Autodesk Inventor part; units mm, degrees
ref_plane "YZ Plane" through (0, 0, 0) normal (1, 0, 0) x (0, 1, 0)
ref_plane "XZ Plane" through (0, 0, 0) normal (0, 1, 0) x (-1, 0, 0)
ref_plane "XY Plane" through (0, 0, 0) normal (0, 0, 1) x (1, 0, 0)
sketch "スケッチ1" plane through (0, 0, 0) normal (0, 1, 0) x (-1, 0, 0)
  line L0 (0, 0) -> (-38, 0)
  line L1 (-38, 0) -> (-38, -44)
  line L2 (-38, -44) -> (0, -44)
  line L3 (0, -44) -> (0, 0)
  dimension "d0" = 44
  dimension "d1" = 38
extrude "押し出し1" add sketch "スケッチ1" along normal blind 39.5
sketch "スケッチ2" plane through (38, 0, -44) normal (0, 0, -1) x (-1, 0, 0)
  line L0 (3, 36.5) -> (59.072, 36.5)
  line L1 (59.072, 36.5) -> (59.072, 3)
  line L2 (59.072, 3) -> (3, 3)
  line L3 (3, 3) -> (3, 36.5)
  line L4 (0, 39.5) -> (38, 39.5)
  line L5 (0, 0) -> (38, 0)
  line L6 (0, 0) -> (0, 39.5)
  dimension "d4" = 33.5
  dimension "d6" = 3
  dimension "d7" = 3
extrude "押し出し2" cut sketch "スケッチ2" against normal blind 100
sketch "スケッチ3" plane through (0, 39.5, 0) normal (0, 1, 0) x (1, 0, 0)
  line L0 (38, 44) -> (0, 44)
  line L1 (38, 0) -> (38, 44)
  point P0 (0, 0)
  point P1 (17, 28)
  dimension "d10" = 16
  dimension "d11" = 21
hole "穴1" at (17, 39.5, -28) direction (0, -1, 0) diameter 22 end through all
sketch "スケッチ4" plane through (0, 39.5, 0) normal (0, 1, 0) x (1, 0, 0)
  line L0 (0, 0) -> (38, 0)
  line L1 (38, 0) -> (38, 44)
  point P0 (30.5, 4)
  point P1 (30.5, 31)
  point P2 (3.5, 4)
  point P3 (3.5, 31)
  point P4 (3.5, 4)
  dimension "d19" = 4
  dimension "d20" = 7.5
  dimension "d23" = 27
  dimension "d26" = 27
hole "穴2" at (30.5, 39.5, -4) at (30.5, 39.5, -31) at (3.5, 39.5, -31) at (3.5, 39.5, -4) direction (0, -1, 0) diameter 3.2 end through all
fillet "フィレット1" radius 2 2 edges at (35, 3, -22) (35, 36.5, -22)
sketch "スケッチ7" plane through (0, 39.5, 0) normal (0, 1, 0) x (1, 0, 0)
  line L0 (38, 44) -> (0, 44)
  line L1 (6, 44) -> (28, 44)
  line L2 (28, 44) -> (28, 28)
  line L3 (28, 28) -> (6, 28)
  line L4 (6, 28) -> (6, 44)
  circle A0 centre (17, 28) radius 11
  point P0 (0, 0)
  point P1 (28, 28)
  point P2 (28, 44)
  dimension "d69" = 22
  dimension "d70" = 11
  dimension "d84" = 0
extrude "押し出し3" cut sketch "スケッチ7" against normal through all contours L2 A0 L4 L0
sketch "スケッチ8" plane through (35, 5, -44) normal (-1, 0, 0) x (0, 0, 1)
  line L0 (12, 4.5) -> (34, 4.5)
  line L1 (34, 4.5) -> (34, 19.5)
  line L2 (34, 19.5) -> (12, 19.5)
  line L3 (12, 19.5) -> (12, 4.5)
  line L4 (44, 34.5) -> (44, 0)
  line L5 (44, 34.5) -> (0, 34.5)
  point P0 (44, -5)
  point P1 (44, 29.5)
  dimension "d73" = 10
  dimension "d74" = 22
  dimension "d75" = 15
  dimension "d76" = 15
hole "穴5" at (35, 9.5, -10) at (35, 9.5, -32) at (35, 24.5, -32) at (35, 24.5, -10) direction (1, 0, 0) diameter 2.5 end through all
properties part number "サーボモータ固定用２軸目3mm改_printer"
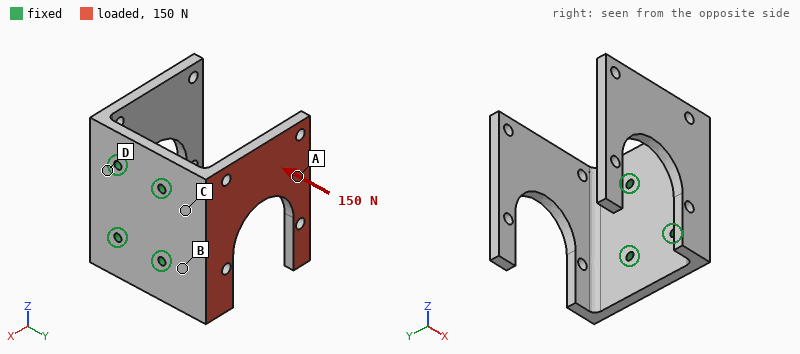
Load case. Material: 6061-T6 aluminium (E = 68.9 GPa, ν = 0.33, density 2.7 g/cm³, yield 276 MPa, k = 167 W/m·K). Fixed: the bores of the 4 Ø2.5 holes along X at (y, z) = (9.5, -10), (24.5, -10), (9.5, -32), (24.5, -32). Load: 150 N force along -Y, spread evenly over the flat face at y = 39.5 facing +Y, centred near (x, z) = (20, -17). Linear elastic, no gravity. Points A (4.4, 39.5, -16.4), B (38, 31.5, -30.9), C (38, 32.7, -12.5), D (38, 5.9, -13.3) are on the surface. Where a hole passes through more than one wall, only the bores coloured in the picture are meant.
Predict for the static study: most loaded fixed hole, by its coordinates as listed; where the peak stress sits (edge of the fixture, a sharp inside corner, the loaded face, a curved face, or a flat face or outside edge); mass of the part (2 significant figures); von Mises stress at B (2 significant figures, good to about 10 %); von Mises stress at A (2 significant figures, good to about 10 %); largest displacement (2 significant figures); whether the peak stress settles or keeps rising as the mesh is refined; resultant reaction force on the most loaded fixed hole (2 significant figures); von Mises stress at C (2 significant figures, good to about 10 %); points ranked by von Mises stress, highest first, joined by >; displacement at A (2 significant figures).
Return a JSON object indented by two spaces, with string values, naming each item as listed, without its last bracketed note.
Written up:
{
  "most loaded fixed hole, by its coordinates as listed": "(24.5, -10)",
  "where the peak stress sits": "edge of the fixture",
  "mass of the part": "30 g",
  "von Mises stress at B": "27 MPa",
  "von Mises stress at A": "17 MPa",
  "largest displacement": "0.54 mm",
  "whether the peak stress settles or keeps rising as the mesh is refined": "keeps rising",
  "resultant reaction force on the most loaded fixed hole": "85 N",
  "von Mises stress at C": "42 MPa",
  "points ranked by von Mises stress, highest first, joined by >": "C > B > A > D",
  "displacement at A": "0.37 mm"
}
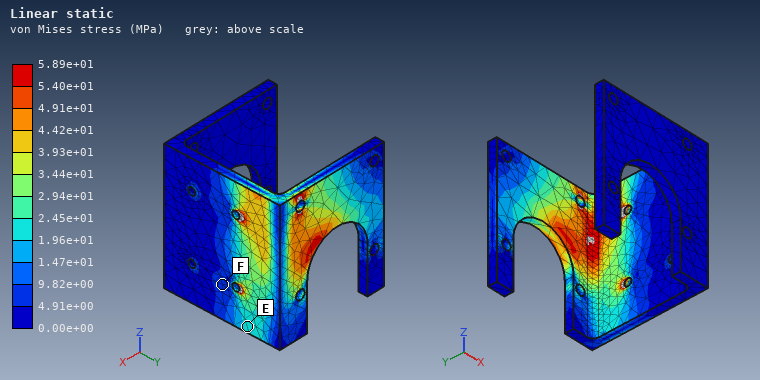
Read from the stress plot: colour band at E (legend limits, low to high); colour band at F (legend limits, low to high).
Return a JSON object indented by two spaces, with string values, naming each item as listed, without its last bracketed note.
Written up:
{
  "colour band at E": "1.96e+01 to 2.45e+01 MPa",
  "colour band at F": "4.91e+00 to 9.82e+00 MPa"
}
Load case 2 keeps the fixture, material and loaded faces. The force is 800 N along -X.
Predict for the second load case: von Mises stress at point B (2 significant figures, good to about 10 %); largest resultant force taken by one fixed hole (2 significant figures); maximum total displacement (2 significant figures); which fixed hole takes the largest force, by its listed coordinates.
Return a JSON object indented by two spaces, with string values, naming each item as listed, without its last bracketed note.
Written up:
{
  "von Mises stress at point B": "84 MPa",
  "largest resultant force taken by one fixed hole": "680 N",
  "maximum total displacement": "0.71 mm",
  "which fixed hole takes the largest force, by its listed coordinates": "(24.5, -10)"
}
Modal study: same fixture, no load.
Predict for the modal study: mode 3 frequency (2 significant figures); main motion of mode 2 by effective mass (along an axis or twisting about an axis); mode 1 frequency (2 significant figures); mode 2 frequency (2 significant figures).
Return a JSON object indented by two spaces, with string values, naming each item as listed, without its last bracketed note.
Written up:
{
  "mode 3 frequency": "2300 Hz",
  "main motion of mode 2 by effective mass": "along Y",
  "mode 1 frequency": "1100 Hz",
  "mode 2 frequency": "1200 Hz"
}
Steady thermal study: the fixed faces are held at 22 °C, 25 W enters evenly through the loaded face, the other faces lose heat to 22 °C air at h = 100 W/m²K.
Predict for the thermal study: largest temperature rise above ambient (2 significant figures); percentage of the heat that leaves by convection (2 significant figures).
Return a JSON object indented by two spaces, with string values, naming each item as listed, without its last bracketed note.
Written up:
{
  "largest temperature rise above ambient": "50 K",
  "percentage of the heat that leaves by convection": "26 %"
}
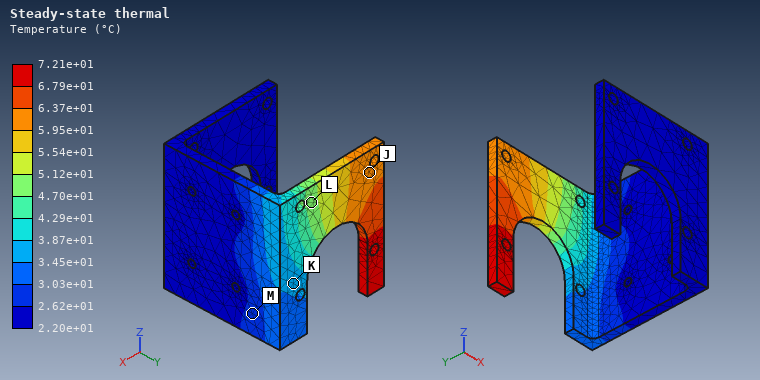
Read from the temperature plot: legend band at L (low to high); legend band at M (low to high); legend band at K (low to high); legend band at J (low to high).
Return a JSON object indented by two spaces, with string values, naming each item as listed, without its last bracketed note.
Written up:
{
  "legend band at L": "4.70e+01 to 5.12e+01 °C",
  "legend band at M": "2.62e+01 to 3.03e+01 °C",
  "legend band at K": "3.45e+01 to 3.87e+01 °C",
  "legend band at J": "5.95e+01 to 6.37e+01 °C"
}
